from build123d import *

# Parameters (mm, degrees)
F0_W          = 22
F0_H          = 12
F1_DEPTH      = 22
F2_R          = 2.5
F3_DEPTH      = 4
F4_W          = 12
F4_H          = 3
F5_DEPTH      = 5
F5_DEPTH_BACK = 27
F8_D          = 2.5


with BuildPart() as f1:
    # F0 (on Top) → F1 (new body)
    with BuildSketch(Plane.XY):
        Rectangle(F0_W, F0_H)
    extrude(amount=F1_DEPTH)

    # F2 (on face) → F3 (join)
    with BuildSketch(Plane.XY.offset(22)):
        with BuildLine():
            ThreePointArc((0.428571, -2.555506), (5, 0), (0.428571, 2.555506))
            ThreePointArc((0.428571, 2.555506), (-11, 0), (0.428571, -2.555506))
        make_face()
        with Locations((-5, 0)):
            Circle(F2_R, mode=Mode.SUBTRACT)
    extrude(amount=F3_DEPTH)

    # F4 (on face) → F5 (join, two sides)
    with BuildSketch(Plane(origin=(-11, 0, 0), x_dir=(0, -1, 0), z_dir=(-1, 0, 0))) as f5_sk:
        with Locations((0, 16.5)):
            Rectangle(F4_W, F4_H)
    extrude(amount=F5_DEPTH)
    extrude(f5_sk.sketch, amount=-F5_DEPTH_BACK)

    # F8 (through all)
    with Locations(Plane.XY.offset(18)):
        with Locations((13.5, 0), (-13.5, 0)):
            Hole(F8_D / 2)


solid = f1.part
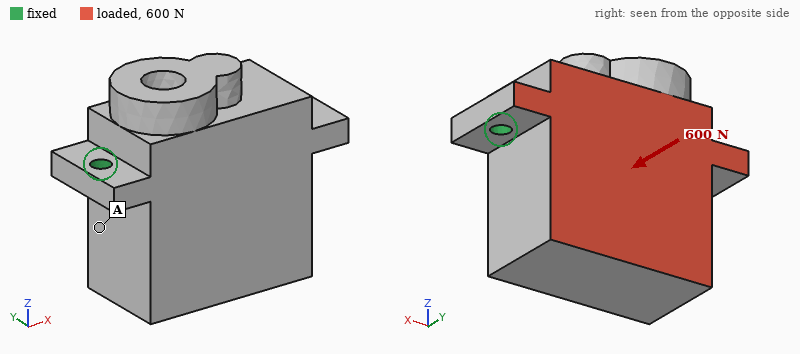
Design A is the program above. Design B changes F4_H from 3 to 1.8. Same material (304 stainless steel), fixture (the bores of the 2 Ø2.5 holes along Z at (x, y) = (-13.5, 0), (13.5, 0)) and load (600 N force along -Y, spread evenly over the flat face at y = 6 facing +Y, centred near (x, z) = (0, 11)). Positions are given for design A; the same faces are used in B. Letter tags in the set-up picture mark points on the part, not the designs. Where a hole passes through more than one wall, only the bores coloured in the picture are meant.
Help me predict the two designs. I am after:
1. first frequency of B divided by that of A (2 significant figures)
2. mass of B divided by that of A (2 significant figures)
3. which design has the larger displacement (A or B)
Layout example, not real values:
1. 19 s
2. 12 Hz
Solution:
1. 0.60
2. 0.98
3. B
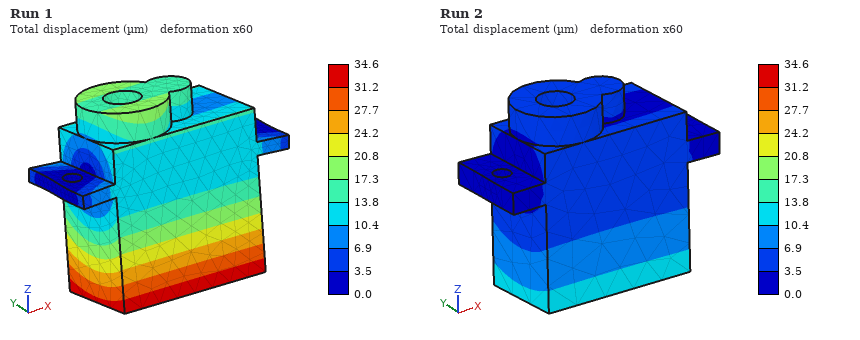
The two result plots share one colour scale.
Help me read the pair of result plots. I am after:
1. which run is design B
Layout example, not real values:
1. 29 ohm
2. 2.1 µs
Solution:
1. Run 1
